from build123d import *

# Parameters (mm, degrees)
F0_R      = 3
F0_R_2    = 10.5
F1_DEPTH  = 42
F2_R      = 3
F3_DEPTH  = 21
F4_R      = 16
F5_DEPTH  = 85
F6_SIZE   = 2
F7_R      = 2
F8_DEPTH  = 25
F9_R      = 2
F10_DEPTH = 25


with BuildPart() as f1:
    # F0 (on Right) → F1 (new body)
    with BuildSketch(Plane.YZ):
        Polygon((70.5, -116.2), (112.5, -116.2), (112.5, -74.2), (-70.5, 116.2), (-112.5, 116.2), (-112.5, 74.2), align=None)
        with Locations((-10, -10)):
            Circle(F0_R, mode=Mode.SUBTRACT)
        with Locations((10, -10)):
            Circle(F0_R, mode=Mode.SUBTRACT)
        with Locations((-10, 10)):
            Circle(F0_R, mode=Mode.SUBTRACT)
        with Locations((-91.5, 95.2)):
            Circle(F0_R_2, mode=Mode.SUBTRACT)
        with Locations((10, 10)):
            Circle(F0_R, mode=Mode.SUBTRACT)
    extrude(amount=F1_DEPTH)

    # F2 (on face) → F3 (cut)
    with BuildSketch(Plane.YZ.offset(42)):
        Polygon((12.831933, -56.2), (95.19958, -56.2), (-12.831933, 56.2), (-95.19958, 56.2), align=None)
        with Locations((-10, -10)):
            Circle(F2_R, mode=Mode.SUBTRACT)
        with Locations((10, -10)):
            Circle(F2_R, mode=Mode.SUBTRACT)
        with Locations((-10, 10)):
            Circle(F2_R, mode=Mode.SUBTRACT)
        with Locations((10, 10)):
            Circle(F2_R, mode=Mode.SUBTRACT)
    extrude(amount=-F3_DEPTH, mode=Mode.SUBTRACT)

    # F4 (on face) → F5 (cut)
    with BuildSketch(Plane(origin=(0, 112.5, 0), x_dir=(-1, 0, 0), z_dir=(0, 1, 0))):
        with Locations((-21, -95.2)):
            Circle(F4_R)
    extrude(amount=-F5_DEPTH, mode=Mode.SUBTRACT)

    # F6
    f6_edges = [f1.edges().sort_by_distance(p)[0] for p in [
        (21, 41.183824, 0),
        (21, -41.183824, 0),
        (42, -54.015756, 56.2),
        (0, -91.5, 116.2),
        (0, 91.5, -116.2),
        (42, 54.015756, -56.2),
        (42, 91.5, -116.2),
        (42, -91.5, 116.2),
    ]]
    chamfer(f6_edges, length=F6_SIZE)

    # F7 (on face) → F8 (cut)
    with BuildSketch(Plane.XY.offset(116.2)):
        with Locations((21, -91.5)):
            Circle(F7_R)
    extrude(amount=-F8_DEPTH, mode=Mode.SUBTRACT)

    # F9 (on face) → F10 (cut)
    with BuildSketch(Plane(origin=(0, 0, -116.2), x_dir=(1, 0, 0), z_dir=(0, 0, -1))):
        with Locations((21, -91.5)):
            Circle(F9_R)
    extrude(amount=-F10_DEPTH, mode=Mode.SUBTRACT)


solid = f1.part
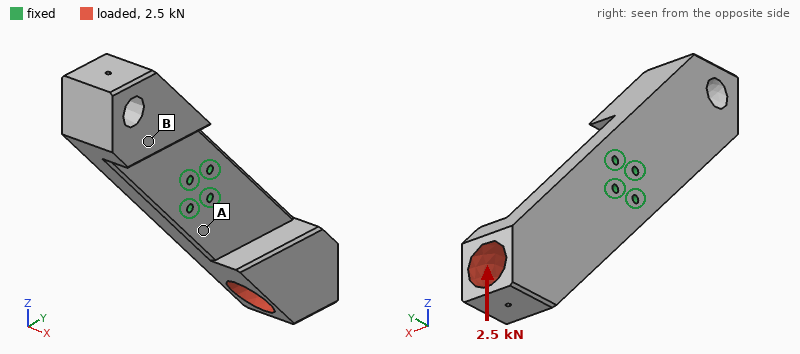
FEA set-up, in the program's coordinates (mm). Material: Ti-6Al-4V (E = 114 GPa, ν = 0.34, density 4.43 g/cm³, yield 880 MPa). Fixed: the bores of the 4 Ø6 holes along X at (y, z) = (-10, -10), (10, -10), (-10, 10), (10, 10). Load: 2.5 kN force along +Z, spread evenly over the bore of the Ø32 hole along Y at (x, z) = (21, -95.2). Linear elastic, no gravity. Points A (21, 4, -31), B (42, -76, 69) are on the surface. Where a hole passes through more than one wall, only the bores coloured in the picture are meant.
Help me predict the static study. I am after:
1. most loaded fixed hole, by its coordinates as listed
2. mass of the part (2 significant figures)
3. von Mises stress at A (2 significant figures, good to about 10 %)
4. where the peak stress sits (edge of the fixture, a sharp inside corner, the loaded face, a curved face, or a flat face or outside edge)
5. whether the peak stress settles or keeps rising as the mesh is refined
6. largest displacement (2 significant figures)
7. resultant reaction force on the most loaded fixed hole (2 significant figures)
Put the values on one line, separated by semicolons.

(10, 10); 2.1 kg; 5.5 MPa; edge of the fixture; keeps rising; 61 µm; 4.4 kN
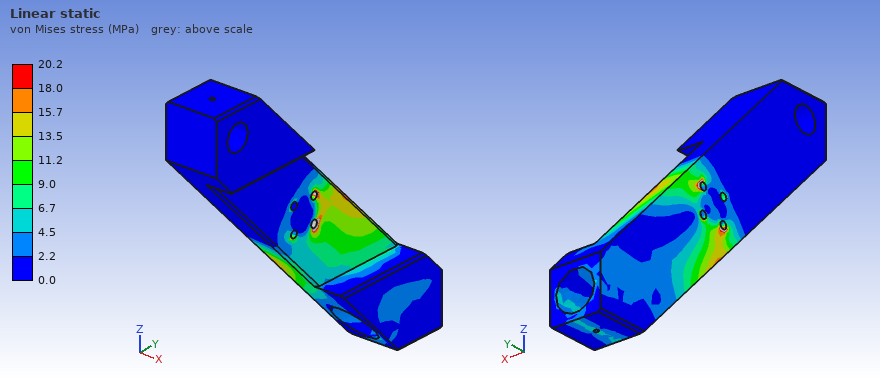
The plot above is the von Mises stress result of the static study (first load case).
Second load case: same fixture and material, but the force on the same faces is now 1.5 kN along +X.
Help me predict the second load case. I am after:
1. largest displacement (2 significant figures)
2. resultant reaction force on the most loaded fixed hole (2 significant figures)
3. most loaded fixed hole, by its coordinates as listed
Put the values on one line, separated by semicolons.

0.21 mm; 3.9 kN; (10, -10)
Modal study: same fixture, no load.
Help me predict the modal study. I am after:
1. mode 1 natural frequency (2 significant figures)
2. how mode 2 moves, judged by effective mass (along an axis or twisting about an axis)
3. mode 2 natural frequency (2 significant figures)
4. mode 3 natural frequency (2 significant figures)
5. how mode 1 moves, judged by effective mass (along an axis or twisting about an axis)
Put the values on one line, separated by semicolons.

690 Hz; along X; 800 Hz; 1400 Hz; along X
